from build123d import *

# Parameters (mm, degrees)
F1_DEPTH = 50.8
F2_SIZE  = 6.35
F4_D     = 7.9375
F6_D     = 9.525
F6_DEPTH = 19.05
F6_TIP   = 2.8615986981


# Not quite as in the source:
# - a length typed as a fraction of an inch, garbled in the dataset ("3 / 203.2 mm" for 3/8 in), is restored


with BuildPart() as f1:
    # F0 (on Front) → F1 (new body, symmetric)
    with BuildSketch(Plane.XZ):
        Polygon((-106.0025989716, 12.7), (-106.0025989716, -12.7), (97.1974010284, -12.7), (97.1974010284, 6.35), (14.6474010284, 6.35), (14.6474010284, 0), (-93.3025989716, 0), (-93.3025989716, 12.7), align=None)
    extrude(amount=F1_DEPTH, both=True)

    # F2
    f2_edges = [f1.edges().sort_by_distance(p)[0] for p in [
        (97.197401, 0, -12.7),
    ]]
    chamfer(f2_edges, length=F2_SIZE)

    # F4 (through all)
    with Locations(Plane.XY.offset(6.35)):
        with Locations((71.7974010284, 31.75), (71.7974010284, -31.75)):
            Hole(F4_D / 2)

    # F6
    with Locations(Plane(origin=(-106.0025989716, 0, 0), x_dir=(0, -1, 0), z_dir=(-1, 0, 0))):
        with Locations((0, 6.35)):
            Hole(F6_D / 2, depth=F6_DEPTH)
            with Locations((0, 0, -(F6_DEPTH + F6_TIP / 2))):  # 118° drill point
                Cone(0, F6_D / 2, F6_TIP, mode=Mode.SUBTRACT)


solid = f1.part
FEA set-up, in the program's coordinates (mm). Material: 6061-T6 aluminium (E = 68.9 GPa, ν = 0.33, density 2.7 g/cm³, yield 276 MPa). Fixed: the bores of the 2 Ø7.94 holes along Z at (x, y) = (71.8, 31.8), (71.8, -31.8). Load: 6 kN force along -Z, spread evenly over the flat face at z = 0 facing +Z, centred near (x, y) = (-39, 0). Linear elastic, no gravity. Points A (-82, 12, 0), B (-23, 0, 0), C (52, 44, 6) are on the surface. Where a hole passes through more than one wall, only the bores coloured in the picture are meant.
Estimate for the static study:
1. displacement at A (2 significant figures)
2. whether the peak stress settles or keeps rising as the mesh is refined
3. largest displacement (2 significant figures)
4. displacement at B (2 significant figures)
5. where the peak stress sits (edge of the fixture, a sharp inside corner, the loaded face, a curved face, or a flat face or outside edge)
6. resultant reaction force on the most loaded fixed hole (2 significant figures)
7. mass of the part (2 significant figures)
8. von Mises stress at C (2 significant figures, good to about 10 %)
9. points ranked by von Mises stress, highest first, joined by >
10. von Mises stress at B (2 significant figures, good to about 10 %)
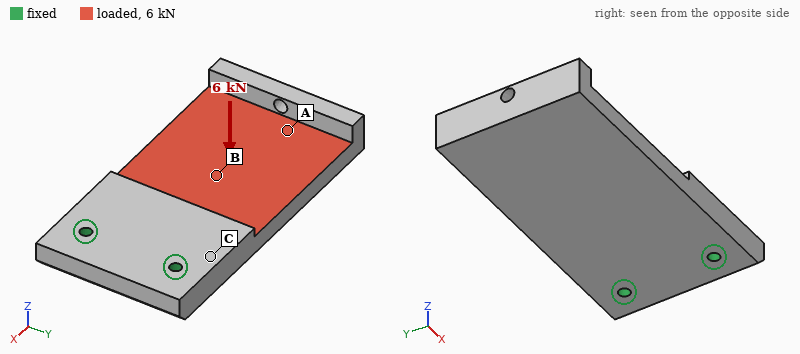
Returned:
1.8 mm
keeps rising
2.2 mm
0.78 mm
edge of the fixture
3.0 kN
880 g
91 MPa
C > B > A
48 MPa
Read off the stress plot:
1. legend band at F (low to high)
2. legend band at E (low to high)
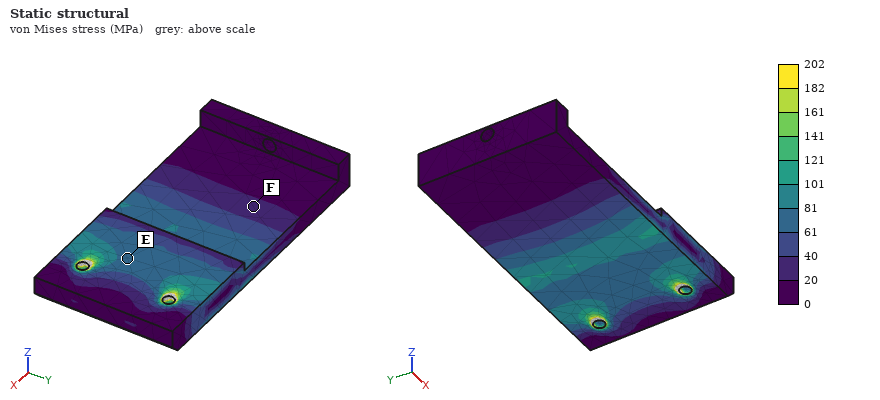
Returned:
20 to 40 MPa
61 to 81 MPa
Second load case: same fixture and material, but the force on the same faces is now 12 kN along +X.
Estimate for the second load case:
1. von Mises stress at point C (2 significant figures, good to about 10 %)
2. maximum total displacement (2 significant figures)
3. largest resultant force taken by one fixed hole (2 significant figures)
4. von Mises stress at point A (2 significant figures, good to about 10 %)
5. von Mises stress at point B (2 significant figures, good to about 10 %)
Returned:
12 MPa
0.40 mm
6.0 kN
4.7 MPa
23 MPa
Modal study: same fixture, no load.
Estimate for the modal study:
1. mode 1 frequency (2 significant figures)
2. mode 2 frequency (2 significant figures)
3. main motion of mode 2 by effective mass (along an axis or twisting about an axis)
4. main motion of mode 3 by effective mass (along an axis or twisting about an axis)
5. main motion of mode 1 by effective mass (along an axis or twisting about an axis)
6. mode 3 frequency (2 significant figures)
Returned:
410 Hz
1300 Hz
twisting about X
along Y
along Z
2100 Hz
